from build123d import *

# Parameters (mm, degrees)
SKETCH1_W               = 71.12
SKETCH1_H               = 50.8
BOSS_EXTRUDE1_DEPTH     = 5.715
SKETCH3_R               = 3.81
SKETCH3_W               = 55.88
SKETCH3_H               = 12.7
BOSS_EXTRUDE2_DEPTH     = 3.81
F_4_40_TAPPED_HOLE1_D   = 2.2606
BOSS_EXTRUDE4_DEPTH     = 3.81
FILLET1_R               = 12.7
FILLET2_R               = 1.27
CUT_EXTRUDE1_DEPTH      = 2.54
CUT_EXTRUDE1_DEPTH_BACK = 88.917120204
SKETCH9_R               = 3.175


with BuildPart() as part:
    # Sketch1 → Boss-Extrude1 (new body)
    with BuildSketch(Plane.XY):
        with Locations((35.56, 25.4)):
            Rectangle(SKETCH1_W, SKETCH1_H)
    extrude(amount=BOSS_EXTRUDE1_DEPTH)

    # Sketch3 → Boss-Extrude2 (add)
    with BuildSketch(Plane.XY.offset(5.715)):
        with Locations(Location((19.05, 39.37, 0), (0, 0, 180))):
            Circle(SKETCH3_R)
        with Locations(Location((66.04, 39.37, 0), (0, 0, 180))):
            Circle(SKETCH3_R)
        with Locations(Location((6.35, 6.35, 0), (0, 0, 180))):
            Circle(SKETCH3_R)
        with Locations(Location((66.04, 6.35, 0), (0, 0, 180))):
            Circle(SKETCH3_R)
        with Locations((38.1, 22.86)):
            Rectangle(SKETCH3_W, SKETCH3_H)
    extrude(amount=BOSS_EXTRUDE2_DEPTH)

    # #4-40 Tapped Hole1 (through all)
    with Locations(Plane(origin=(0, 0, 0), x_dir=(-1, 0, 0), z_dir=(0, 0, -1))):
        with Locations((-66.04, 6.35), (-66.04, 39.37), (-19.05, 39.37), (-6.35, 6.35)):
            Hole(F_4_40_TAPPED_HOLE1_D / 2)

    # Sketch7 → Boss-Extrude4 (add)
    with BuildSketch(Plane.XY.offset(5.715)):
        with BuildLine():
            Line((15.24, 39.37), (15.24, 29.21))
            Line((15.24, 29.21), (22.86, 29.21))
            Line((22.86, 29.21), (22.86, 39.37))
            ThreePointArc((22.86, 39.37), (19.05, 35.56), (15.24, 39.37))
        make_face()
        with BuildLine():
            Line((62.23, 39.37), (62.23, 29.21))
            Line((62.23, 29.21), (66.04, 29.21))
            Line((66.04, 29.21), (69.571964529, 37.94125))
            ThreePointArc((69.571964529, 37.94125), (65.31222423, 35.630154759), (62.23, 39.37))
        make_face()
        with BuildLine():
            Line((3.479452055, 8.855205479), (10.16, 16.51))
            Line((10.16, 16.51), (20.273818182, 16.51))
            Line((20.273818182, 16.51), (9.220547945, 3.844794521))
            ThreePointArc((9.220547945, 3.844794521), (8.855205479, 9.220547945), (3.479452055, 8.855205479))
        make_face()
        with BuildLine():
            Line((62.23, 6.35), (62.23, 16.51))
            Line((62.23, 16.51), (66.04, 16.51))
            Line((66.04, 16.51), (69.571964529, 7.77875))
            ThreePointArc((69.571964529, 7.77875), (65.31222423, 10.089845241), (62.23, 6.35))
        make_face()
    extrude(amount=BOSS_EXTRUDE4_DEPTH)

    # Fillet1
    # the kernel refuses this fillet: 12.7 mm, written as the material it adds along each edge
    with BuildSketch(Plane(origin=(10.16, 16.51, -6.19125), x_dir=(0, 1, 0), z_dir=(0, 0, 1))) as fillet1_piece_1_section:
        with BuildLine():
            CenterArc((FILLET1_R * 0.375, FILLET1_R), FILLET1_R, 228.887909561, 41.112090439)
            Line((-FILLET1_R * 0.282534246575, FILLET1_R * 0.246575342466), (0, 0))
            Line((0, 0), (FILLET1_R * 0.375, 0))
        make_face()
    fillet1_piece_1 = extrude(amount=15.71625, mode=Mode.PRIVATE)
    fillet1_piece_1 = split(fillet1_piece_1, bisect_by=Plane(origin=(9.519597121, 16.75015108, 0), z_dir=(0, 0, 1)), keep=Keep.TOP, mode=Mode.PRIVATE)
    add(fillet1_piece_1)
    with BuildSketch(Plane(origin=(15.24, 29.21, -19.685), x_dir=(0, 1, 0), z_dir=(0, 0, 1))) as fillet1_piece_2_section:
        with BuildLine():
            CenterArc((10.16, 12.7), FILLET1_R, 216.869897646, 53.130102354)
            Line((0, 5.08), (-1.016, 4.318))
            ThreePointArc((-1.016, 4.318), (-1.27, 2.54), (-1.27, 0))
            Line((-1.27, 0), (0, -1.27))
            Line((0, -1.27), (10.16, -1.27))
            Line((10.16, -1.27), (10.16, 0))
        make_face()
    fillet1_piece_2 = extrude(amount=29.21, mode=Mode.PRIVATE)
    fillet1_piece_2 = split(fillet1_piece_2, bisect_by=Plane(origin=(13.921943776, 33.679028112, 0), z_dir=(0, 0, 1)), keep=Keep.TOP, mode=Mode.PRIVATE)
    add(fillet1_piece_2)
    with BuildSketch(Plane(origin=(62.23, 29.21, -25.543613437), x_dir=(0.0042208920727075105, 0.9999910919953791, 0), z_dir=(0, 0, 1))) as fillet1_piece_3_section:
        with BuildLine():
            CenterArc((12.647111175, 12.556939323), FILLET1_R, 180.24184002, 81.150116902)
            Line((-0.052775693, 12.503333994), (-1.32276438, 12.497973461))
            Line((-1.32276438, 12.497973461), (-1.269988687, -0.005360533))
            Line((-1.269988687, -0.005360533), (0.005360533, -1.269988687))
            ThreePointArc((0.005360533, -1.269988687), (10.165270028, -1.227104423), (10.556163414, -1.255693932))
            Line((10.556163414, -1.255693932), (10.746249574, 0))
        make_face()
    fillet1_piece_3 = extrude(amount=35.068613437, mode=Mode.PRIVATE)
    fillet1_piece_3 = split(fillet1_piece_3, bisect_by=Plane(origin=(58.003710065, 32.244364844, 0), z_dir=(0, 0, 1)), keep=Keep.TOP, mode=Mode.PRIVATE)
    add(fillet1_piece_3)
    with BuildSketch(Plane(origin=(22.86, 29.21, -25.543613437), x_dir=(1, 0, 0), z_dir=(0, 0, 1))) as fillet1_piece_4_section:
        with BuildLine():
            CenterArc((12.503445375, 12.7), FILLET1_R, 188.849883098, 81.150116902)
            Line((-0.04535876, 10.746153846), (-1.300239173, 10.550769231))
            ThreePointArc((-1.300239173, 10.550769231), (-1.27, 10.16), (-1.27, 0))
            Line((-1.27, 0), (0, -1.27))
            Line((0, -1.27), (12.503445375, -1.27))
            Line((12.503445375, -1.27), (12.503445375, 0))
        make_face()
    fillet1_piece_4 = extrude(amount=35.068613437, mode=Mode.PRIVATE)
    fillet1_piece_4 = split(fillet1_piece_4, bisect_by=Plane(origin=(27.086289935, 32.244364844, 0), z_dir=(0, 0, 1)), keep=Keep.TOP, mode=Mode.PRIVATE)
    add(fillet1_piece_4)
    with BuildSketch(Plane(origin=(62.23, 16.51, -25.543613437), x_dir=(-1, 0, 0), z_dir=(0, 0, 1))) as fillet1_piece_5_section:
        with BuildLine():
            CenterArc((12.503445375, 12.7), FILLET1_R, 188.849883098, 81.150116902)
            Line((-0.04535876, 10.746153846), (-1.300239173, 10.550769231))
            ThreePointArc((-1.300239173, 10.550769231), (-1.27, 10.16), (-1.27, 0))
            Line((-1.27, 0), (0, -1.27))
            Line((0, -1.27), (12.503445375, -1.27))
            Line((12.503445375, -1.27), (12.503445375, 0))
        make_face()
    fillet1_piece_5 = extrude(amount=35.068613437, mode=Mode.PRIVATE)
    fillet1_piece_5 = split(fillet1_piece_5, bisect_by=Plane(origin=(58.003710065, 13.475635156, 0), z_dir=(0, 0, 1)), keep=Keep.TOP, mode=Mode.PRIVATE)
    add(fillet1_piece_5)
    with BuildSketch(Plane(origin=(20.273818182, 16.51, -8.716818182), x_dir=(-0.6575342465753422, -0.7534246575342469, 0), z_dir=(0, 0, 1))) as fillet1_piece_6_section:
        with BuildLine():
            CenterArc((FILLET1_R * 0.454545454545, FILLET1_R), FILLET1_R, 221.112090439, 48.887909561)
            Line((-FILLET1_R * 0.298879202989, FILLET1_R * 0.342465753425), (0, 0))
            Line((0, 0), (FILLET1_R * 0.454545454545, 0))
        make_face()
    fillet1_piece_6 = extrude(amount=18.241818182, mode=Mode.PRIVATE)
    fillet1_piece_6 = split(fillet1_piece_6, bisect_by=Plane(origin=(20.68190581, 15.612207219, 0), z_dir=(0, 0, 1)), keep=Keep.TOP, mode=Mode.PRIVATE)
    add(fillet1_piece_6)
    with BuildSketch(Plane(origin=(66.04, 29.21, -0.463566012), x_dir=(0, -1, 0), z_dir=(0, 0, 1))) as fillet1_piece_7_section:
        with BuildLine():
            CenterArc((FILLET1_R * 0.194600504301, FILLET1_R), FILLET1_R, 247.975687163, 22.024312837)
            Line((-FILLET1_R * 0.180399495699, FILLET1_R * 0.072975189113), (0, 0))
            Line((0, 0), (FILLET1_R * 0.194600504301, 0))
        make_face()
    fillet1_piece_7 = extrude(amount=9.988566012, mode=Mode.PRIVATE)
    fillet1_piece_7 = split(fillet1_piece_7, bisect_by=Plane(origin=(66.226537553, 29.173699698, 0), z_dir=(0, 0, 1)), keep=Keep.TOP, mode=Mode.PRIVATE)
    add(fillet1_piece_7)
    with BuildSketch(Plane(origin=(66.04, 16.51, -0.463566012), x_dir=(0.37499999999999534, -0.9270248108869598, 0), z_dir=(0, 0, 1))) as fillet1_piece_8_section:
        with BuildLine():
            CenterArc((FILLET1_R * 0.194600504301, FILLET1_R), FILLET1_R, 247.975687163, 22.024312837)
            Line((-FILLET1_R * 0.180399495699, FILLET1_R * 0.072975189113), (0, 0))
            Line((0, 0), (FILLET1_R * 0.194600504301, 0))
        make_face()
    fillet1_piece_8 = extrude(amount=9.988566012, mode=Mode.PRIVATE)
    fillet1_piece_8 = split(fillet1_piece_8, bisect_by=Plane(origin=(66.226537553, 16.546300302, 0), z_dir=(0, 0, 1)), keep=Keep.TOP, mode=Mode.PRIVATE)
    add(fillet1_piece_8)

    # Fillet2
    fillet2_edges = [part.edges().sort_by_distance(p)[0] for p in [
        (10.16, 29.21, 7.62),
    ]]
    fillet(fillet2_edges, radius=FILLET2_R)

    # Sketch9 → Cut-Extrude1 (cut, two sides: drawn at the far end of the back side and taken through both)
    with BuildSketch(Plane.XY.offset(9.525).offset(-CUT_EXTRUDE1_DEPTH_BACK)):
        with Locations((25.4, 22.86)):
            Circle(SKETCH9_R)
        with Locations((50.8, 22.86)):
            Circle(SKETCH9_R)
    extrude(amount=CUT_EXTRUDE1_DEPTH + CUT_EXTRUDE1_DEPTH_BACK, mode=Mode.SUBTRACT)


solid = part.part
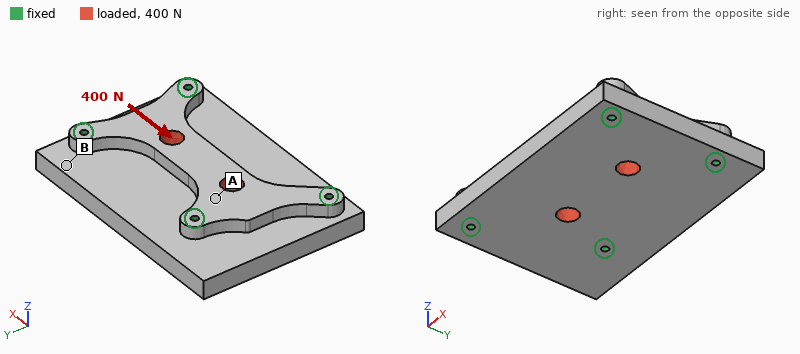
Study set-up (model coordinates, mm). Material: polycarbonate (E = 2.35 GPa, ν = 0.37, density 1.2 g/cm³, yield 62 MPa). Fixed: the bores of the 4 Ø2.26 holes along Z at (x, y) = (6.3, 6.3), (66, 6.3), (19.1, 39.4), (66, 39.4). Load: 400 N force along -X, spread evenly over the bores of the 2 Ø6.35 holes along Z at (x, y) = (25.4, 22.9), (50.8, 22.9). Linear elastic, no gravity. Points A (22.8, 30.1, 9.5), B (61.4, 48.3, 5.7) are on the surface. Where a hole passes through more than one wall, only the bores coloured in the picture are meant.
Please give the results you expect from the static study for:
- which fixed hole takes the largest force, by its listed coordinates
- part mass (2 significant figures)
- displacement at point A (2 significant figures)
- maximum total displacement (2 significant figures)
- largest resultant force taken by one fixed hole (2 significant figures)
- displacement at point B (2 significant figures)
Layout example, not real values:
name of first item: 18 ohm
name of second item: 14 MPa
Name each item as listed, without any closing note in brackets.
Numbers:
which fixed hole takes the largest force, by its listed coordinates: (19.1, 39.4)
part mass: 29 g
displacement at point A: 8.8 µm
maximum total displacement: 15 µm
largest resultant force taken by one fixed hole: 120 N
displacement at point B: 2.9 µm
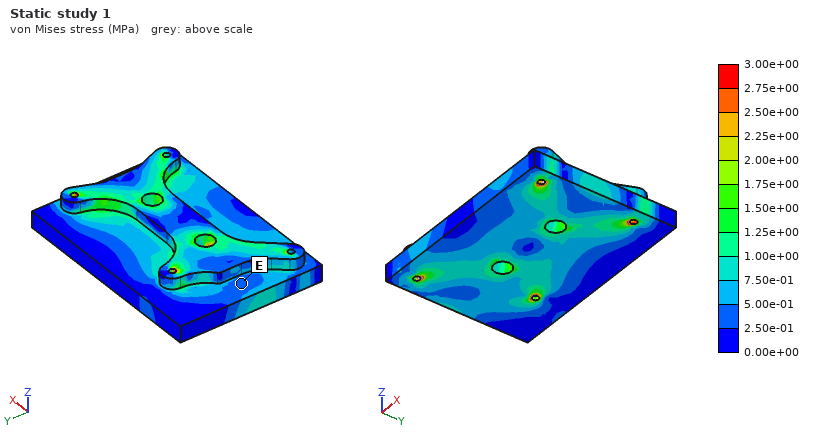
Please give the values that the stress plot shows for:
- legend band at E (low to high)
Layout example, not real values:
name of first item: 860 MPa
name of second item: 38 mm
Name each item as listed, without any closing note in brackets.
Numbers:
legend band at E: 2.50e-01 to 5.00e-01 MPa
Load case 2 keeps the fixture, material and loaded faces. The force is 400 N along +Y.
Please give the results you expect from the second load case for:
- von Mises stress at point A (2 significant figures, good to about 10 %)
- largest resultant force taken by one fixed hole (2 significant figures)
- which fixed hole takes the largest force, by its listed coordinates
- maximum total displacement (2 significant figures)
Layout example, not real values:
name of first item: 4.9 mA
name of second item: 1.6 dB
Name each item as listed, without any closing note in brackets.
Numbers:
von Mises stress at point A: 1.5 MPa
largest resultant force taken by one fixed hole: 170 N
which fixed hole takes the largest force, by its listed coordinates: (19.1, 39.4)
maximum total displacement: 19 µm
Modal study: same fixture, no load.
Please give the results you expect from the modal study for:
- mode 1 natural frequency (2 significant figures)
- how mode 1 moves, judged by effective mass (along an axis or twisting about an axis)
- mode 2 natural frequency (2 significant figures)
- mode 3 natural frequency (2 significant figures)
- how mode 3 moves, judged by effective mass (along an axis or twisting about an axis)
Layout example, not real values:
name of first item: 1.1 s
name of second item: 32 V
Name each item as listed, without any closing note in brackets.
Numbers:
mode 1 natural frequency: 2600 Hz
how mode 1 moves, judged by effective mass: along Z
mode 2 natural frequency: 3500 Hz
mode 3 natural frequency: 3900 Hz
how mode 3 moves, judged by effective mass: along Z
